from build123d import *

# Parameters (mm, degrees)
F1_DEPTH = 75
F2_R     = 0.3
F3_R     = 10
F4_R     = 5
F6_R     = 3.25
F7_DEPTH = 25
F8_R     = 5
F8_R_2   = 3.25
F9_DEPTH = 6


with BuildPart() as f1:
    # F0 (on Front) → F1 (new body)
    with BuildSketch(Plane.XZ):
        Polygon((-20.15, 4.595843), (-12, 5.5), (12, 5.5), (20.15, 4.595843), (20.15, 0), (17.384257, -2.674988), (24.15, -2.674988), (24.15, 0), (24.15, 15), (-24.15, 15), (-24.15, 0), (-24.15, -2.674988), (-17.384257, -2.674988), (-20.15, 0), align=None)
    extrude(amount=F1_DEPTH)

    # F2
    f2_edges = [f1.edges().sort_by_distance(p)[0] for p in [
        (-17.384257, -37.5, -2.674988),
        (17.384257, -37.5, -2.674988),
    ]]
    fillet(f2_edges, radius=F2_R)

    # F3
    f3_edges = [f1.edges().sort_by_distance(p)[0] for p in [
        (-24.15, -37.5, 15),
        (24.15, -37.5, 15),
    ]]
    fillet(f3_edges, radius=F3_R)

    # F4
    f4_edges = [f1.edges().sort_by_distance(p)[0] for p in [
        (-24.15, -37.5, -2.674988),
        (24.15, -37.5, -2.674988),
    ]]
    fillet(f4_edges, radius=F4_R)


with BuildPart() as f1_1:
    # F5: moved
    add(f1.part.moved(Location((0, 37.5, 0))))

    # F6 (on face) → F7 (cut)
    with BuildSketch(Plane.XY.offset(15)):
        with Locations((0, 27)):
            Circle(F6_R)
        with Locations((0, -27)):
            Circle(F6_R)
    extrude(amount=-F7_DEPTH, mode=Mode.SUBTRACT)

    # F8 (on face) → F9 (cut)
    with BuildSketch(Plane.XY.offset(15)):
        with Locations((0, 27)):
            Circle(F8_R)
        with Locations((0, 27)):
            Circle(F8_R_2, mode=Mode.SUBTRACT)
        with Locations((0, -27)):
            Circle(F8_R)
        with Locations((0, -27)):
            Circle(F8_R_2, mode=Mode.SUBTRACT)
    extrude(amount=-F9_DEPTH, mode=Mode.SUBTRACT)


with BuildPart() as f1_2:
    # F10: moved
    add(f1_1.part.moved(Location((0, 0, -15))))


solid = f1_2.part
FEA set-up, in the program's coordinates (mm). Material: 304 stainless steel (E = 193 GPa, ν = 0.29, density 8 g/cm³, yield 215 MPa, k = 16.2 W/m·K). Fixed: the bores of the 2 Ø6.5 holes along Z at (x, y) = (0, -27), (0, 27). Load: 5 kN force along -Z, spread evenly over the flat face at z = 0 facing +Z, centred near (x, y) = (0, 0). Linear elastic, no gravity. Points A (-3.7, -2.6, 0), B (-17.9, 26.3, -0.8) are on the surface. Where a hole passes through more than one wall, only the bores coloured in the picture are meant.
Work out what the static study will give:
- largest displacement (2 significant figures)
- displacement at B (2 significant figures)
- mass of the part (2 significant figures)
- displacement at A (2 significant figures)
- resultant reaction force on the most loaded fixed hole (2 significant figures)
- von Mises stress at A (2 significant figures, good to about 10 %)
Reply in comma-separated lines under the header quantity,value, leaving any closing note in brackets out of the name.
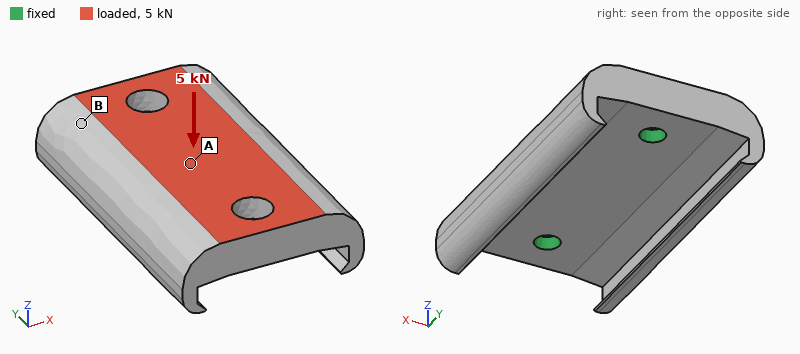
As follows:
quantity,value
largest displacement,7.7 µm
displacement at B,4.2 µm
mass of the part,280 g
displacement at A,6.9 µm
resultant reaction force on the most loaded fixed hole,2.6 kN
von Mises stress at A,19 MPa
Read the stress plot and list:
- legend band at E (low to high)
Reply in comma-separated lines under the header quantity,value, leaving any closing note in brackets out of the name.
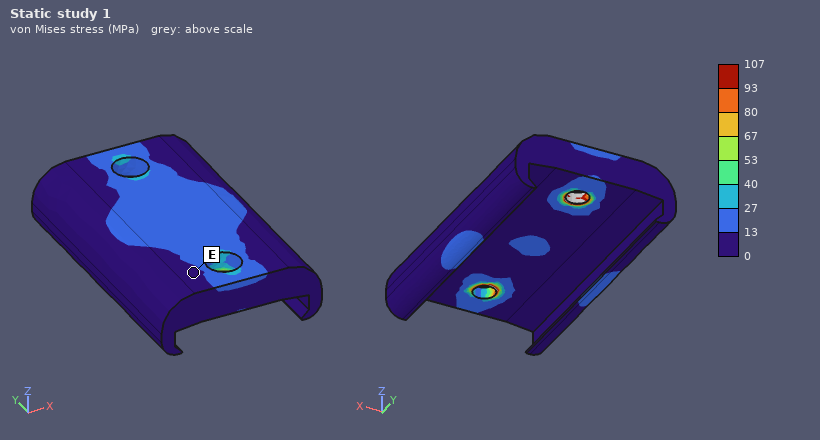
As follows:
quantity,value
legend band at E,0 to 13 MPa
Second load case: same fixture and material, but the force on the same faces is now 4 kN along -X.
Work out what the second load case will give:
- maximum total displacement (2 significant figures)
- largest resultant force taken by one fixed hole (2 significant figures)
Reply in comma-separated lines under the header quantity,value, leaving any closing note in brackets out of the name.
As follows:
quantity,value
maximum total displacement,23 µm
largest resultant force taken by one fixed hole,2.0 kN
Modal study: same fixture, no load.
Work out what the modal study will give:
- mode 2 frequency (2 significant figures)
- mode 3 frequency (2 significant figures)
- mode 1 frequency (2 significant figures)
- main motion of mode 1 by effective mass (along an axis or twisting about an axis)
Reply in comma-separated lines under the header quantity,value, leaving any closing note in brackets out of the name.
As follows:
quantity,value
mode 2 frequency,7700 Hz
mode 3 frequency,8000 Hz
mode 1 frequency,3600 Hz
main motion of mode 1 by effective mass,twisting about Y
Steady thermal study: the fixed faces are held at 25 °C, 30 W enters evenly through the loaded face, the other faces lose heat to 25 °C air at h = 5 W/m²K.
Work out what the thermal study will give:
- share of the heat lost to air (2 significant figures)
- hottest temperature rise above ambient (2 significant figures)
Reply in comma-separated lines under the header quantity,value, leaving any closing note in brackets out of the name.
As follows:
quantity,value
share of the heat lost to air,6.7 %
hottest temperature rise above ambient,58 K
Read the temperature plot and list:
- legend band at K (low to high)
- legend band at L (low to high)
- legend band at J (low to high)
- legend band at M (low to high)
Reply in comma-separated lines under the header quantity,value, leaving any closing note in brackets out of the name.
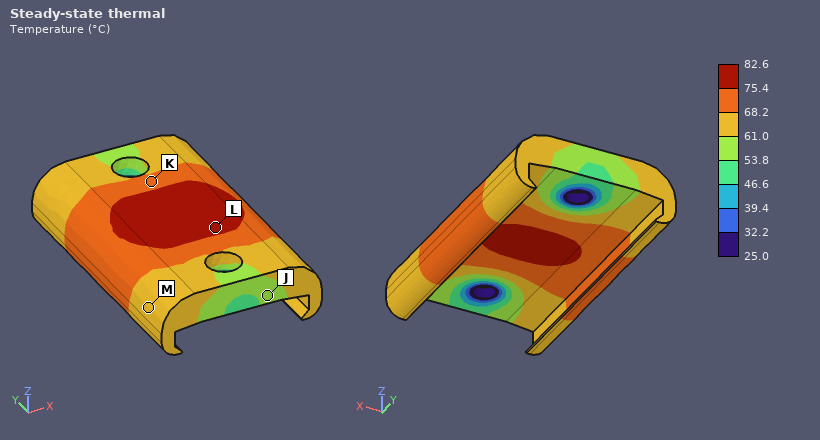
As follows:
quantity,value
legend band at K,68.2 to 75.4 °C
legend band at L,75.4 to 82.6 °C
legend band at J,53.8 to 61.0 °C
legend band at M,61.0 to 68.2 °C
